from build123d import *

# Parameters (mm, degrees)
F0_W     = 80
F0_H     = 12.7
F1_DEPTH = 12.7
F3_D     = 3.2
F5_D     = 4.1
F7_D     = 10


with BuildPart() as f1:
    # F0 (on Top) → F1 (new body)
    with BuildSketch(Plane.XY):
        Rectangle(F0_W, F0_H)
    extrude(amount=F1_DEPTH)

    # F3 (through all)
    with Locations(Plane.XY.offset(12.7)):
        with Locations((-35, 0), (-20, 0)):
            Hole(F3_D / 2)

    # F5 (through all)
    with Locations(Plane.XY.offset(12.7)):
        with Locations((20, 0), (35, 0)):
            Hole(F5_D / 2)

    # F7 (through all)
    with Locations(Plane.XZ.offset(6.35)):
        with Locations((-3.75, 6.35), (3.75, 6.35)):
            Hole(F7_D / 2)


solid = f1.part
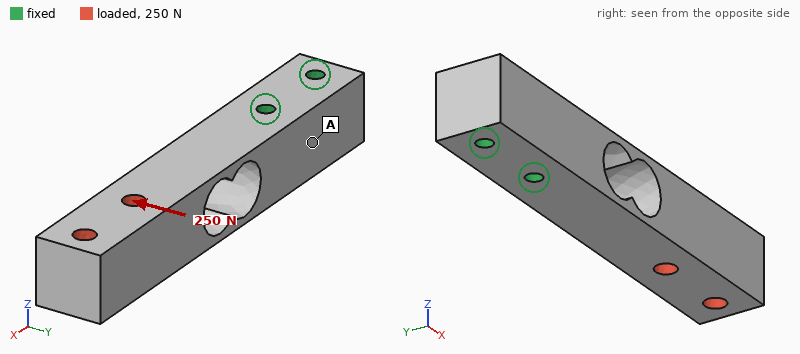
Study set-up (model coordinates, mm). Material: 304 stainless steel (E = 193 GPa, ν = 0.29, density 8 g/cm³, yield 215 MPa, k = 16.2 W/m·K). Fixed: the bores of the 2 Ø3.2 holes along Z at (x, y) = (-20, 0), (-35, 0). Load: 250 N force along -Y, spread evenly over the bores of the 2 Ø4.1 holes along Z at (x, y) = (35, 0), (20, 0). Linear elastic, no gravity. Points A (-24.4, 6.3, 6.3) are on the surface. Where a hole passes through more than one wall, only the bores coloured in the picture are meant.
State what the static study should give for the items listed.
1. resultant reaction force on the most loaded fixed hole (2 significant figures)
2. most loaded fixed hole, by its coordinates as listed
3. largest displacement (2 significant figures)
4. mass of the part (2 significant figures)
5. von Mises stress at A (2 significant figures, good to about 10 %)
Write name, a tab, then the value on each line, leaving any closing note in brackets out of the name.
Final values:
resultant reaction force on the most loaded fixed hole	740 N
most loaded fixed hole, by its coordinates as listed	(-20, 0)
largest displacement	82 µm
mass of the part	84 g
von Mises stress at A	16 MPa
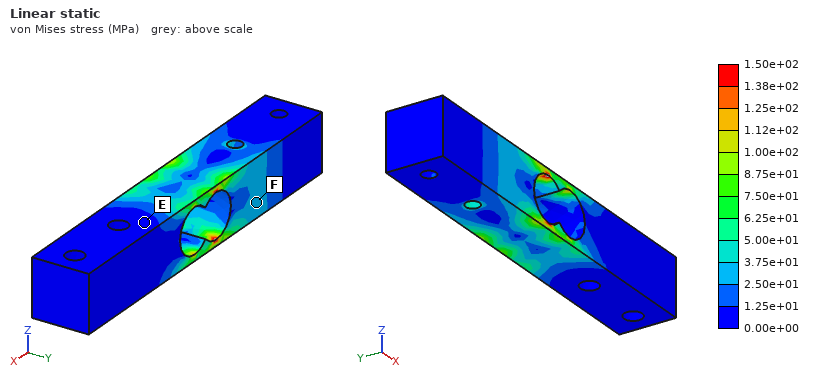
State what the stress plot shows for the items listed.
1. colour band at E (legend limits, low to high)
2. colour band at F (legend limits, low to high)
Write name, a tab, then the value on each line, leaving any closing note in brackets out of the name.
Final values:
colour band at E	0.00e+00 to 1.25e+01 MPa
colour band at F	2.50e+01 to 3.75e+01 MPa
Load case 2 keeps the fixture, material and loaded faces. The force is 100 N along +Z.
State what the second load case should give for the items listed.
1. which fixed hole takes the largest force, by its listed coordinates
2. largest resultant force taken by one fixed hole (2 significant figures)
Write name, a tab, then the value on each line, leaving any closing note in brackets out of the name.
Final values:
which fixed hole takes the largest force, by its listed coordinates	(-20, 0)
largest resultant force taken by one fixed hole	150 N
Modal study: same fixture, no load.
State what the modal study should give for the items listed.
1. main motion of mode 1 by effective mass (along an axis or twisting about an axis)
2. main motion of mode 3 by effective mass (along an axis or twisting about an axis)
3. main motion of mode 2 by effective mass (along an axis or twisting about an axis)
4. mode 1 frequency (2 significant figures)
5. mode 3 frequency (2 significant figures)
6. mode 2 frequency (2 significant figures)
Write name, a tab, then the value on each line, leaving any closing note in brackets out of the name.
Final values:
main motion of mode 1 by effective mass	along Z
main motion of mode 3 by effective mass	twisting about X
main motion of mode 2 by effective mass	along Y
mode 1 frequency	1600 Hz
mode 3 frequency	6800 Hz
mode 2 frequency	1800 Hz
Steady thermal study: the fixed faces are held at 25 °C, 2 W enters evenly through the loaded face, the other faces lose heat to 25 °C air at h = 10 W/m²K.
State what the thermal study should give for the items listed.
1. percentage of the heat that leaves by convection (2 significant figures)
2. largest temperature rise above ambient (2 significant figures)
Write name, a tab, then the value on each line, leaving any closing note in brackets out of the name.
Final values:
percentage of the heat that leaves by convection	46 %
largest temperature rise above ambient	45 K
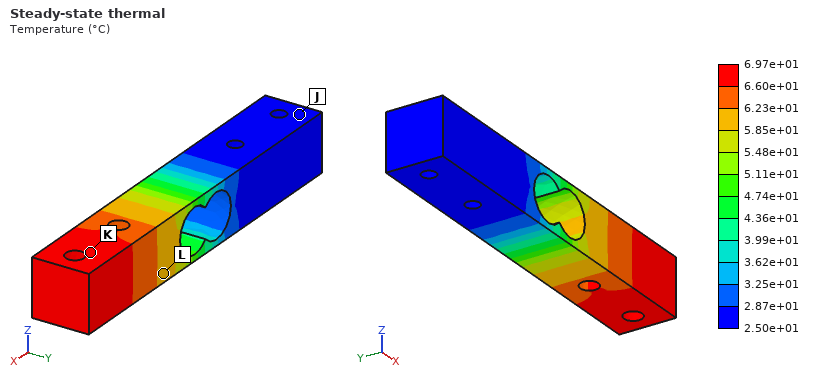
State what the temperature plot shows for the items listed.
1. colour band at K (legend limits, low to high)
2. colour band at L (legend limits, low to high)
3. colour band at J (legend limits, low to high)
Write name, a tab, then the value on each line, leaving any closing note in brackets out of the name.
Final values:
colour band at K	6.60e+01 to 6.97e+01 °C
colour band at L	5.85e+01 to 6.23e+01 °C
colour band at J	2.50e+01 to 2.87e+01 °C
